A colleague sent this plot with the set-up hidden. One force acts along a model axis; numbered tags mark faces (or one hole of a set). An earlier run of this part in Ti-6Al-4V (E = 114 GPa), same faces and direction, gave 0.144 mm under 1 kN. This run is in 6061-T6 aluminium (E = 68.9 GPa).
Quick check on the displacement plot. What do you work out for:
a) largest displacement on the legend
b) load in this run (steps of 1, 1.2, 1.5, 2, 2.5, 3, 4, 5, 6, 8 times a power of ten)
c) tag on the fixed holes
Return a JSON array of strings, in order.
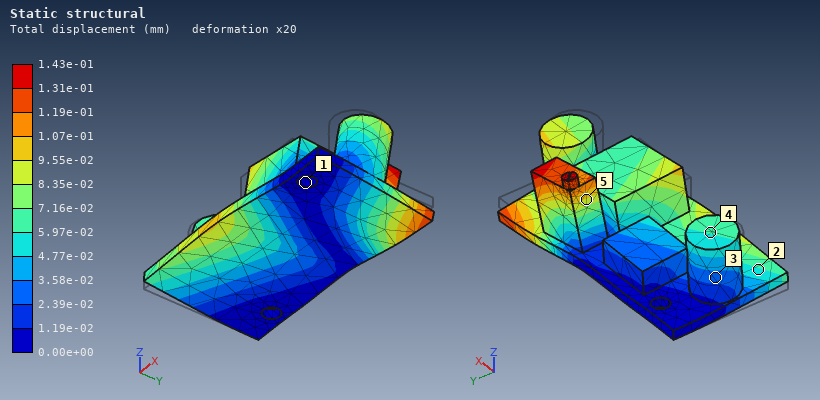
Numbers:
["1.43e-01 mm", "600 N", "1"]
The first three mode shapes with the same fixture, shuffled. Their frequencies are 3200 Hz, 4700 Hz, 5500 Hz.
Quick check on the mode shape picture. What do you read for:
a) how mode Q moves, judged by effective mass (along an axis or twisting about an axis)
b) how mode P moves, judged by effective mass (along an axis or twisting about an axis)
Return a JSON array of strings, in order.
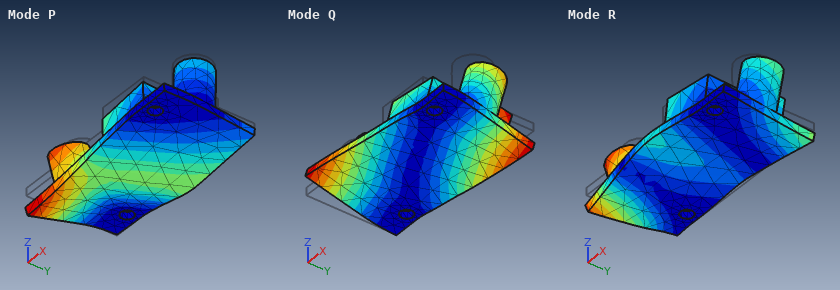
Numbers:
["along Y", "along Z"]
